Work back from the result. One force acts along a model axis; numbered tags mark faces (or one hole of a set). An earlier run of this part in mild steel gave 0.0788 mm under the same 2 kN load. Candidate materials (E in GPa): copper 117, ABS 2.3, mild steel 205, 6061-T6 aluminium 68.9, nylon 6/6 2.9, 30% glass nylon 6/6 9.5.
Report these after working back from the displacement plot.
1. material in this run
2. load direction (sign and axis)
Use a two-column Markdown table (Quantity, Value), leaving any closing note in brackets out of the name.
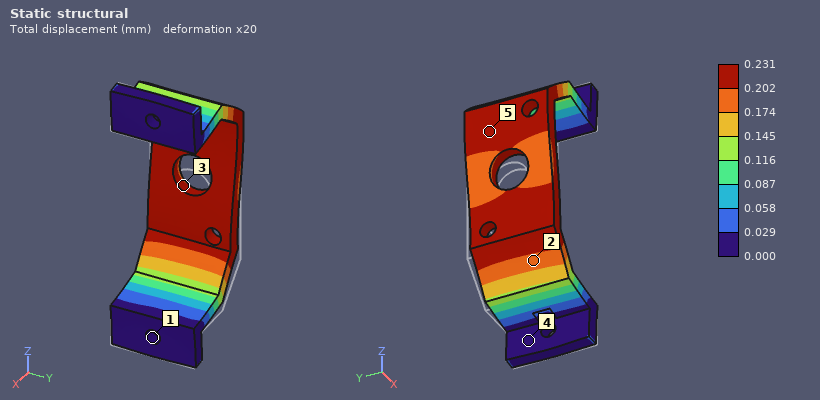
| Quantity | Value |
|---|---|
| material in this run | 6061-T6 aluminium |
| load direction | +Z |
